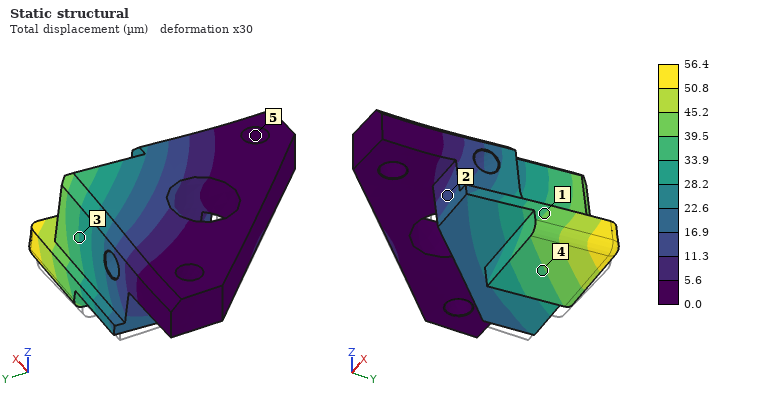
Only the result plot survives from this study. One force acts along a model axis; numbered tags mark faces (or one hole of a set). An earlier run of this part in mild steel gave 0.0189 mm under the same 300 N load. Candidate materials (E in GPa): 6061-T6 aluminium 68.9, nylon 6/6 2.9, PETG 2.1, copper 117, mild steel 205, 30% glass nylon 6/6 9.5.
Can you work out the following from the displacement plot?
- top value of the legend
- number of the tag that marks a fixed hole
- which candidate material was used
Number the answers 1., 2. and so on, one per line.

1. 56.4 µm
2. 5
3. 6061-T6 aluminium
